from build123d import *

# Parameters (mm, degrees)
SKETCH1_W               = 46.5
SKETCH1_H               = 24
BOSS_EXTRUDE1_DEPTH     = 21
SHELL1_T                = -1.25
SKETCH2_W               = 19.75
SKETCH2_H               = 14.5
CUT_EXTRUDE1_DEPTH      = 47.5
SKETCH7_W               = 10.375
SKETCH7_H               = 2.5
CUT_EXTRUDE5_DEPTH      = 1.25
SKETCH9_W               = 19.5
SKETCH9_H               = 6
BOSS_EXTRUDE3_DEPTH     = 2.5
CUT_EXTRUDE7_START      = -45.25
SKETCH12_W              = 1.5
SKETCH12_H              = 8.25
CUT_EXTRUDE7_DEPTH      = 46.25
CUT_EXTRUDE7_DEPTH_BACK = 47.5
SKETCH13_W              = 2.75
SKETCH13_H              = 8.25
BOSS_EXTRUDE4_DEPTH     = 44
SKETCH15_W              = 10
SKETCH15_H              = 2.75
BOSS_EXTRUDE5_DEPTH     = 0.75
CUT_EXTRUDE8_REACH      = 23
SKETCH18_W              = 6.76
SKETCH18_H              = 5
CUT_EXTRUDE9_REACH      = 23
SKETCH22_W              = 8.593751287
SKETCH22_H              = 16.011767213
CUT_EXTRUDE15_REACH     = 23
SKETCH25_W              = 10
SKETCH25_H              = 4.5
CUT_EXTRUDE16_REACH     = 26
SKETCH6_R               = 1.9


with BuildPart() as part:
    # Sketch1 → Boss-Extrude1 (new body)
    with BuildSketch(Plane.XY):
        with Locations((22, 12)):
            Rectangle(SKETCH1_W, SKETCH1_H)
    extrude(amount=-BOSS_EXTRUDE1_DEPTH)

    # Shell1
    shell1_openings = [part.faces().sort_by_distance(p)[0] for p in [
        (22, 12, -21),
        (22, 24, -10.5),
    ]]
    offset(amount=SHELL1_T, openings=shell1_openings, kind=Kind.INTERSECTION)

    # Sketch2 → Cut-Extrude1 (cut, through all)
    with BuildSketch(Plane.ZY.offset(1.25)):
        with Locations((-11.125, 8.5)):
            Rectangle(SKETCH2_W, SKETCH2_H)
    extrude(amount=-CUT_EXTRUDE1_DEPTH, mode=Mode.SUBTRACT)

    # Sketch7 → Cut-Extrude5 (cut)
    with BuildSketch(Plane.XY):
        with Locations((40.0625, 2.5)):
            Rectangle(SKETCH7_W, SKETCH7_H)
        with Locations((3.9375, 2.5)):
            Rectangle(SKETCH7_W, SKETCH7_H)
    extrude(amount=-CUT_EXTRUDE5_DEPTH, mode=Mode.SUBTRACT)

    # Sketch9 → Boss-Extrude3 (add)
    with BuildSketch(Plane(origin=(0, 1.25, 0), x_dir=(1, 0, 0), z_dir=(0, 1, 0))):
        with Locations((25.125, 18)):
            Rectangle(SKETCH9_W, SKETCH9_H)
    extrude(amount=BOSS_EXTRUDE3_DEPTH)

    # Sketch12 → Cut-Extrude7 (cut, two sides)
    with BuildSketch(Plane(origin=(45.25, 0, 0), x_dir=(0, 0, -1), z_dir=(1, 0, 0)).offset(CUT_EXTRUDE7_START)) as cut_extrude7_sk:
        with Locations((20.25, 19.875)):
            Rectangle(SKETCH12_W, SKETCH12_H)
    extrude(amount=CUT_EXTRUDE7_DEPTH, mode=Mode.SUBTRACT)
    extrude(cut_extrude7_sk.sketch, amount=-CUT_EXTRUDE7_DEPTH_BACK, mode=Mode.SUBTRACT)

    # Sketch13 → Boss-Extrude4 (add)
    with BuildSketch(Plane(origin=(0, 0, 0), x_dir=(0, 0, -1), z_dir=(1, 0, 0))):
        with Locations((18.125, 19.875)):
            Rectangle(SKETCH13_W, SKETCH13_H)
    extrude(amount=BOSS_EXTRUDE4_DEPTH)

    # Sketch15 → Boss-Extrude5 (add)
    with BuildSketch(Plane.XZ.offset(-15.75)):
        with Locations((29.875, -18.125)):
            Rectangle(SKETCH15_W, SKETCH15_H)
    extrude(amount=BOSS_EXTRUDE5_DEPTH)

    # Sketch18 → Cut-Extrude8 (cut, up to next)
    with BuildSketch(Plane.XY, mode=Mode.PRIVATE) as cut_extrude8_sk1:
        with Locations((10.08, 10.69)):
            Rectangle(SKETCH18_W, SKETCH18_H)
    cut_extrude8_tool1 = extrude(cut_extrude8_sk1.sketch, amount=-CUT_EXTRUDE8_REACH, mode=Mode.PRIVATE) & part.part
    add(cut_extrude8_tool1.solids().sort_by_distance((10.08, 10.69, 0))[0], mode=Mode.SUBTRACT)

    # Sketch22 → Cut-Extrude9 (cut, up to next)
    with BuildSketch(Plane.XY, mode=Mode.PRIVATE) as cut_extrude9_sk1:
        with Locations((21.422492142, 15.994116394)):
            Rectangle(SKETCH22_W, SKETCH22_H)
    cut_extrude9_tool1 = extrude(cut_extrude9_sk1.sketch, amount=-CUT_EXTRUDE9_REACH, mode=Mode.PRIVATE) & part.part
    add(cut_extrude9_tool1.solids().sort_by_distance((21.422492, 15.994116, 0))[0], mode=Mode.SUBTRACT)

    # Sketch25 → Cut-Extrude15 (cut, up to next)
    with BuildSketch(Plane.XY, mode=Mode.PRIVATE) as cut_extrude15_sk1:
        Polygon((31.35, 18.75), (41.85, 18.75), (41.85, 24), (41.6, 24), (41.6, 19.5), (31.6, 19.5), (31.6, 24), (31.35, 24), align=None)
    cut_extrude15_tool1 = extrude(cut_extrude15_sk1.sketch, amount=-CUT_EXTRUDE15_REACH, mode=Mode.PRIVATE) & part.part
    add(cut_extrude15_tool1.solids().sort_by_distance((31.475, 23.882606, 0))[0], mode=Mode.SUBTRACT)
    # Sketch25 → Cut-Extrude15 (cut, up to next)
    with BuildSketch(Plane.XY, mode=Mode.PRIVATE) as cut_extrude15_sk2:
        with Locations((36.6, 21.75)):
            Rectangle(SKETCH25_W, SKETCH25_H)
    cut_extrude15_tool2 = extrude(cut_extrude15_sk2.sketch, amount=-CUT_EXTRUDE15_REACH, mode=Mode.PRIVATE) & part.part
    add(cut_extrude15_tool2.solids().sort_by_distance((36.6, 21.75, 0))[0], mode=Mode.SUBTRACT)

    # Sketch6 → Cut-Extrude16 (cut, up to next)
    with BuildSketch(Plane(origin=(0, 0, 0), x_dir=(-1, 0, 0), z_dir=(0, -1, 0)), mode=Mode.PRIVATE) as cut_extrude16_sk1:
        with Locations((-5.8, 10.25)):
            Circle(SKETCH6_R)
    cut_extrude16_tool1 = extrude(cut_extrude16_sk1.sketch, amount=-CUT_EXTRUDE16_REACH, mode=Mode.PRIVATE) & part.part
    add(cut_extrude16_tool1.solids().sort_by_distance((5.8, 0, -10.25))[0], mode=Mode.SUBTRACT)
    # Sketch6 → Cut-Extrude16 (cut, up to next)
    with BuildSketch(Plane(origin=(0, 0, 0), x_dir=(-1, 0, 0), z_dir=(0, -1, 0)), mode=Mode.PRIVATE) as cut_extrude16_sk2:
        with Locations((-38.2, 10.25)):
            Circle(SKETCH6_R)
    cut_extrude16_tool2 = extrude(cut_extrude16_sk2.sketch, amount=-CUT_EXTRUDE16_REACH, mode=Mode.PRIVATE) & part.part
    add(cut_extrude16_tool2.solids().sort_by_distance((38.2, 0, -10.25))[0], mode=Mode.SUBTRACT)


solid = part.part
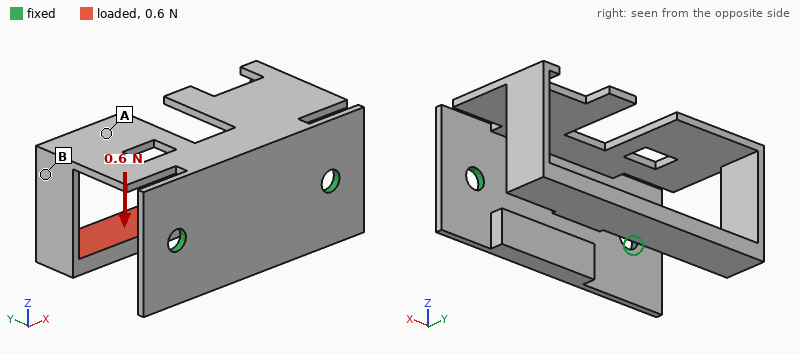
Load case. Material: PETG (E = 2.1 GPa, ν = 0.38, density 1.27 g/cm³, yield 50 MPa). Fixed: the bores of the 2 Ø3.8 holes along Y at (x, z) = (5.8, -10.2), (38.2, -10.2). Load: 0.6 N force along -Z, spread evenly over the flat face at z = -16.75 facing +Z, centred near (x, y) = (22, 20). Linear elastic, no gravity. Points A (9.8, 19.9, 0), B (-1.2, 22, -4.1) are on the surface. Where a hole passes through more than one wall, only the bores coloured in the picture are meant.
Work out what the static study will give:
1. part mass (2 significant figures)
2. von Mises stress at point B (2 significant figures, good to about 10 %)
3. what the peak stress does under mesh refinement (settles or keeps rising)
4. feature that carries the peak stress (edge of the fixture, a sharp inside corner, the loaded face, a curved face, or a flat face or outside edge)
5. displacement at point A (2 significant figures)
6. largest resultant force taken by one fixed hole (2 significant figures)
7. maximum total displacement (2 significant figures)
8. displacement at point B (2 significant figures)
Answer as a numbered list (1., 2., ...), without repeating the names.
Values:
1. 4.9 g
2. 0.63 MPa
3. keeps rising
4. a sharp inside corner
5. 0.35 mm
6. 0.31 N
7. 0.65 mm
8. 0.46 mm
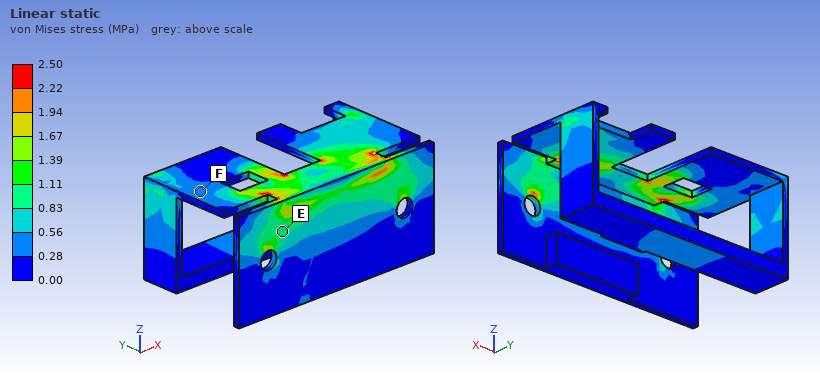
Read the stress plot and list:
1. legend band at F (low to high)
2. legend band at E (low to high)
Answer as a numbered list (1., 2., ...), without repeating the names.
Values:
1. 0.28 to 0.56 MPa
2. 0.83 to 1.11 MPa
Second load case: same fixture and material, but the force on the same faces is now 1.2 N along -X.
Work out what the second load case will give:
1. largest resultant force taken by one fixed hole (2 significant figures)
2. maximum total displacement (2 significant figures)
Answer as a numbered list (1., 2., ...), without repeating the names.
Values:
1. 1.1 N
2. 0.66 mm
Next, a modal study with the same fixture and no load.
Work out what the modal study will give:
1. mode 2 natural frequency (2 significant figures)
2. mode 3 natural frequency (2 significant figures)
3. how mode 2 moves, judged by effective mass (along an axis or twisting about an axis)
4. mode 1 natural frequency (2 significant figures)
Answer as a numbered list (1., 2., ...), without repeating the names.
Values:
1. 160 Hz
2. 270 Hz
3. along X
4. 100 Hz
